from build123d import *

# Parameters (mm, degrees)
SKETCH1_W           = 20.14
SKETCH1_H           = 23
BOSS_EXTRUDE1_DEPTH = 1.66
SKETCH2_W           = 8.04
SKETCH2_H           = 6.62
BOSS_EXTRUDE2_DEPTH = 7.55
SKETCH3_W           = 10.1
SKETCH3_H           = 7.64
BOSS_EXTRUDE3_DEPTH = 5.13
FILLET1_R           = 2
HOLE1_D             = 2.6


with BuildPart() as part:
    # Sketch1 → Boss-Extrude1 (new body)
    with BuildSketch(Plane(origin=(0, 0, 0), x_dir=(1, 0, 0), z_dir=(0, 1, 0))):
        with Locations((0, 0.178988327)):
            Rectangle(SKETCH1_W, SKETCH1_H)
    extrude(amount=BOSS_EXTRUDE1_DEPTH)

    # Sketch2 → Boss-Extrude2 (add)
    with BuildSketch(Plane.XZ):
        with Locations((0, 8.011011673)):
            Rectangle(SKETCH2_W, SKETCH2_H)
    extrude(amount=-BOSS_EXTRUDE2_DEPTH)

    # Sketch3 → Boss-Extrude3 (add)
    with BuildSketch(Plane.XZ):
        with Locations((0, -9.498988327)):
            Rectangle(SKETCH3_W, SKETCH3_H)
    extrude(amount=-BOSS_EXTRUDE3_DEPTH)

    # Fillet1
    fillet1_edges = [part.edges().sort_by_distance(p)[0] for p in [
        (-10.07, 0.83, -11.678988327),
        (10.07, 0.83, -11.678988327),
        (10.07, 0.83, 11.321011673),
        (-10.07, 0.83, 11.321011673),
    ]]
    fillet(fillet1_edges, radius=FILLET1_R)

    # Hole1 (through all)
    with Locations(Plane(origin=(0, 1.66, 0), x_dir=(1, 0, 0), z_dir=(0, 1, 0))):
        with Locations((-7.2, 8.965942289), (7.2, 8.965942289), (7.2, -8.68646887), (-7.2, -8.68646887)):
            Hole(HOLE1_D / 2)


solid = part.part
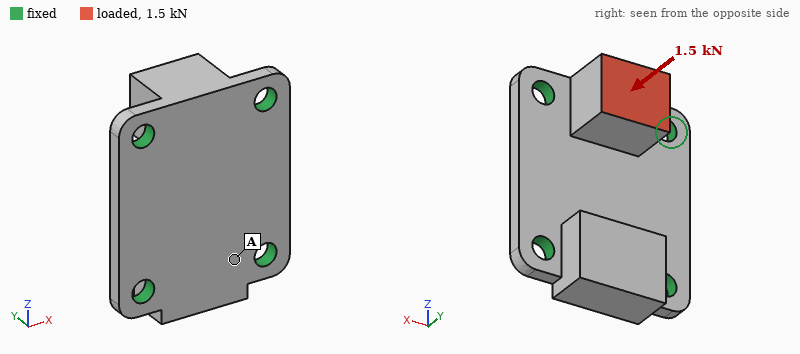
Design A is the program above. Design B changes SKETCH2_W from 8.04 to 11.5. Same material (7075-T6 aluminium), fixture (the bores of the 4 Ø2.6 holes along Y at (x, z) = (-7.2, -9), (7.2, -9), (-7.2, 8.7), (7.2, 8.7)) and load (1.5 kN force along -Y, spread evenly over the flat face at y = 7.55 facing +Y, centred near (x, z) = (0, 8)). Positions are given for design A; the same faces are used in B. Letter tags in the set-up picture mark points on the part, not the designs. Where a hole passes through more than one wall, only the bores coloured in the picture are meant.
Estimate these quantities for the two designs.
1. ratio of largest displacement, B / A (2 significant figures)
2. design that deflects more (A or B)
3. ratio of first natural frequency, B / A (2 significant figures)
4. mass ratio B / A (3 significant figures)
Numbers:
0.53
A
1.1
1.10
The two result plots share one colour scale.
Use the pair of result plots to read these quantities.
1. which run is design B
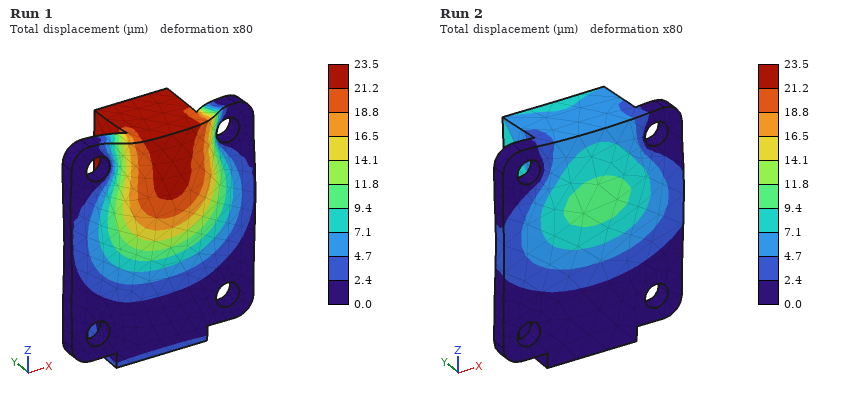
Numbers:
Run 2
